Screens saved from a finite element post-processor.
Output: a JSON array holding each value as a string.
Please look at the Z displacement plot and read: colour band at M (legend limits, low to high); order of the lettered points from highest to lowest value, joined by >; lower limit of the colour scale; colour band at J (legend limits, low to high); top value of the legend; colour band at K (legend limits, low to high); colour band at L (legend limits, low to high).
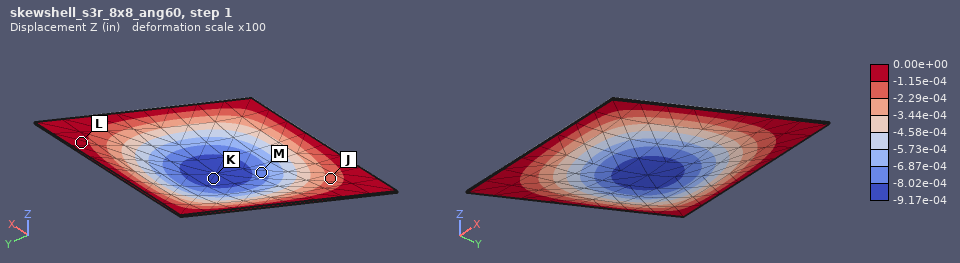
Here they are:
["-8.02e-04 to -6.87e-04 in", "L > J > M > K", "-9.17e-04 in", "-2.29e-04 to -1.15e-04 in", "0.00e+00 in", "-9.17e-04 to -8.02e-04 in", "-1.15e-04 to 0.00e+00 in"]
